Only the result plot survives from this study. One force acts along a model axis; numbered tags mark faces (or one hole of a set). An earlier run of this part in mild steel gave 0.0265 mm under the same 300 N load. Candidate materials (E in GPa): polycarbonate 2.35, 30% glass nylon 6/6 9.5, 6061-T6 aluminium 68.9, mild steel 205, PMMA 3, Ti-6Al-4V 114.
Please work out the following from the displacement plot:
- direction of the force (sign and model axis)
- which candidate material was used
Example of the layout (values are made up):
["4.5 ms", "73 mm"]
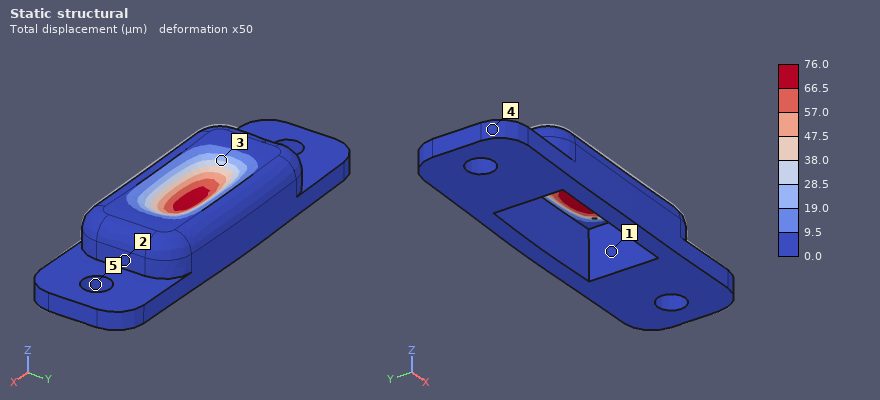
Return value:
["-Z", "6061-T6 aluminium"]
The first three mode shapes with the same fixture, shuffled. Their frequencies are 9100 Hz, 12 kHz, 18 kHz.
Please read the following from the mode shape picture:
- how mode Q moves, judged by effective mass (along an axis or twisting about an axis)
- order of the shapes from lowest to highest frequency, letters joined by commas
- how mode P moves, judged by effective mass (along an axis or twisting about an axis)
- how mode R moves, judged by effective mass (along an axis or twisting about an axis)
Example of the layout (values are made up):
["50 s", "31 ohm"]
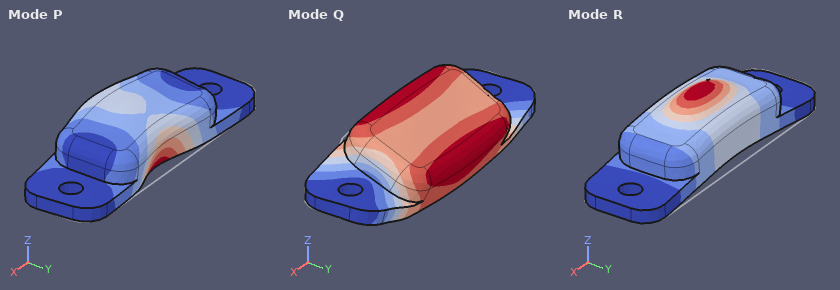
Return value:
["along Y", "Q, R, P", "along Y", "along Z"]
